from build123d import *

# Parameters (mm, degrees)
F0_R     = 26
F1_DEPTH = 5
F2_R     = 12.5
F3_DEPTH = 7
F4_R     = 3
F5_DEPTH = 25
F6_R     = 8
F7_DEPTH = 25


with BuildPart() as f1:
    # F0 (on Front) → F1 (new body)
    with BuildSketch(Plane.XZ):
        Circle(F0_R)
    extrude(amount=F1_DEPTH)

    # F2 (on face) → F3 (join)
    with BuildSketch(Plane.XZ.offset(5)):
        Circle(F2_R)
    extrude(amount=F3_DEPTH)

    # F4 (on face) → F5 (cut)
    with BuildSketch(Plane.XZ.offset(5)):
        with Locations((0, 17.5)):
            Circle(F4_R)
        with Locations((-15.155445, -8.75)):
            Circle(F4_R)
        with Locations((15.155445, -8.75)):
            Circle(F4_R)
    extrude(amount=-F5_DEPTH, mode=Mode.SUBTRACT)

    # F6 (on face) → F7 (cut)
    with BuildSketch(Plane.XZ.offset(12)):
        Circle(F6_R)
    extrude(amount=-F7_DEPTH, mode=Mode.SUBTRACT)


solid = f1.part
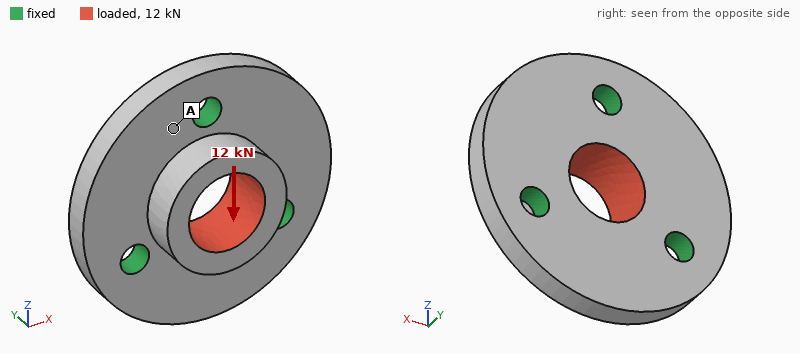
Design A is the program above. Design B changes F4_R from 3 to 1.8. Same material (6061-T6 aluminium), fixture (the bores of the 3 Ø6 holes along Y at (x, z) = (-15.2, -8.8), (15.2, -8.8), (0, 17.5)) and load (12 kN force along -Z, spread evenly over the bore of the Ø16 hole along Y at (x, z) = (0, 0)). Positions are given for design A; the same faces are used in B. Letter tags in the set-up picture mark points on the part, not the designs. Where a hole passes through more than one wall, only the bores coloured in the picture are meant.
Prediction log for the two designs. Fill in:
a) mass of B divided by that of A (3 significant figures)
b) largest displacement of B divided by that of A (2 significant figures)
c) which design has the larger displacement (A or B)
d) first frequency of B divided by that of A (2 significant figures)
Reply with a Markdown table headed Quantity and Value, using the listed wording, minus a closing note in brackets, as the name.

| Quantity | Value |
|---|---|
| mass of B divided by that of A | 1.02 |
| largest displacement of B divided by that of A | 1.2 |
| which design has the larger displacement | B |
| first frequency of B divided by that of A | 0.84 |
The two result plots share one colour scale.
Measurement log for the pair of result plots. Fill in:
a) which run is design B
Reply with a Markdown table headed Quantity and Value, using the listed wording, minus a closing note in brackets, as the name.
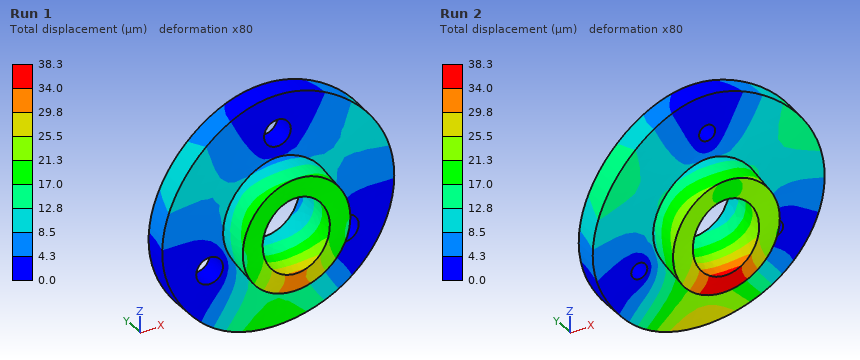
| Quantity | Value |
|---|---|
| which run is design B | Run 2 |
